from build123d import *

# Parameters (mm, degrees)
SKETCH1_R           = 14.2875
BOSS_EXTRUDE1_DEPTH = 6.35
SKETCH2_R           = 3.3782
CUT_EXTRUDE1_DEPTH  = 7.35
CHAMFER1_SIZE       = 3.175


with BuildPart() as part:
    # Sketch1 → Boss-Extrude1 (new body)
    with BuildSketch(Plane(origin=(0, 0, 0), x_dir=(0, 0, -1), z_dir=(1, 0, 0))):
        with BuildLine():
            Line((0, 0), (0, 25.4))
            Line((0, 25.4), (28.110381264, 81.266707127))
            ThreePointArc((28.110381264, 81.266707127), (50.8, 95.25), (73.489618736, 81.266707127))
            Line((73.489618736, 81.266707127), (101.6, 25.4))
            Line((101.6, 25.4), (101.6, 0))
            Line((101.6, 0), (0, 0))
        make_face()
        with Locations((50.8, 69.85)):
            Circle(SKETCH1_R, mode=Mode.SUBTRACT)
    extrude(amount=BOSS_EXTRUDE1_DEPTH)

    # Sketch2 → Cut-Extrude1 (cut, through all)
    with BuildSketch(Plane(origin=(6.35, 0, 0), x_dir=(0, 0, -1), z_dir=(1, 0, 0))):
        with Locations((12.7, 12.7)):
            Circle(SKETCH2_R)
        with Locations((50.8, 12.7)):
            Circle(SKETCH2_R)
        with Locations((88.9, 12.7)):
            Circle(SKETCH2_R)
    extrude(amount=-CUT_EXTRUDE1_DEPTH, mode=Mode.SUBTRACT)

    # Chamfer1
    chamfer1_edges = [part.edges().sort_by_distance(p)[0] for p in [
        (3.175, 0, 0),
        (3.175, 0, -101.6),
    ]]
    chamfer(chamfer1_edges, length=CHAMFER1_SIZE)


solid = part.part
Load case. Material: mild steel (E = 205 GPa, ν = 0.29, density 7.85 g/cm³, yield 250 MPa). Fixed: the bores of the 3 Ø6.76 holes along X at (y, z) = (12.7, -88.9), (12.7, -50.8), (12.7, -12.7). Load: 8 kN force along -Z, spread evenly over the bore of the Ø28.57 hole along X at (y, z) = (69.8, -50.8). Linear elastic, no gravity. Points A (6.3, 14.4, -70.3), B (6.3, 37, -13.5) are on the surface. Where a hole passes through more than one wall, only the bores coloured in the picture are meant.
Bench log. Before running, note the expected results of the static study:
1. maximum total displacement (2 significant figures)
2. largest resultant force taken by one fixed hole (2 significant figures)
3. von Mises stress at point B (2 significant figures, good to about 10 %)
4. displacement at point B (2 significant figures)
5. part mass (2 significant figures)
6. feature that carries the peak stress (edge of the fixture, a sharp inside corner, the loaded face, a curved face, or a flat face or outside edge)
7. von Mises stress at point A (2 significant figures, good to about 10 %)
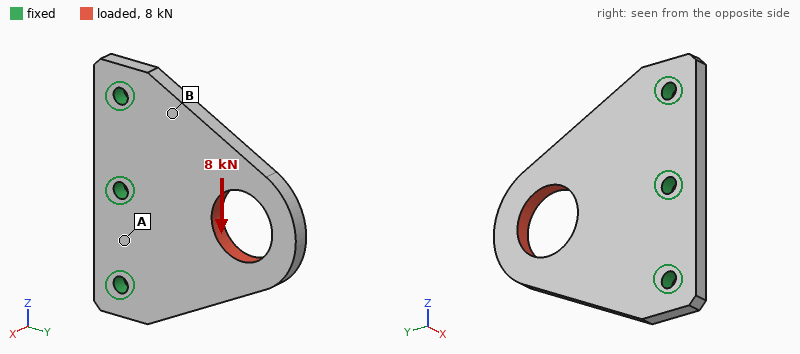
37 µm
6.3 kN
36 MPa
7.0 µm
320 g
edge of the fixture
12 MPa
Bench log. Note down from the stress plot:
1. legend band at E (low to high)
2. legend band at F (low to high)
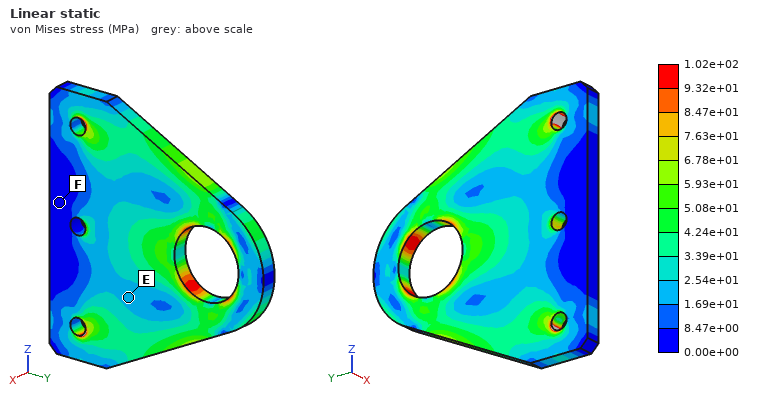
1.69e+01 to 2.54e+01 MPa
0.00e+00 to 8.47e+00 MPa
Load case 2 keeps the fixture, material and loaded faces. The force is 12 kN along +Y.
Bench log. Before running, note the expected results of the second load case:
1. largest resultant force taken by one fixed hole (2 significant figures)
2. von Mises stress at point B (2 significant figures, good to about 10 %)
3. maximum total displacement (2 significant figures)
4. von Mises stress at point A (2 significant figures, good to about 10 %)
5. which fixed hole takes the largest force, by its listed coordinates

4.7 kN
21 MPa
17 µm
7.5 MPa
(12.7, -50.8)
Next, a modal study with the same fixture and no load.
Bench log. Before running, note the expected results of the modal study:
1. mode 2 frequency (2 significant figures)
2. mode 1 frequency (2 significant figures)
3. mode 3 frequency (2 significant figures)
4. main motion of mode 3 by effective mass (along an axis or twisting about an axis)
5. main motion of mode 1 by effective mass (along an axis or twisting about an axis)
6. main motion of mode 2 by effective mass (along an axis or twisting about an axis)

3300 Hz
1200 Hz
4700 Hz
along X
along X
twisting about Y
